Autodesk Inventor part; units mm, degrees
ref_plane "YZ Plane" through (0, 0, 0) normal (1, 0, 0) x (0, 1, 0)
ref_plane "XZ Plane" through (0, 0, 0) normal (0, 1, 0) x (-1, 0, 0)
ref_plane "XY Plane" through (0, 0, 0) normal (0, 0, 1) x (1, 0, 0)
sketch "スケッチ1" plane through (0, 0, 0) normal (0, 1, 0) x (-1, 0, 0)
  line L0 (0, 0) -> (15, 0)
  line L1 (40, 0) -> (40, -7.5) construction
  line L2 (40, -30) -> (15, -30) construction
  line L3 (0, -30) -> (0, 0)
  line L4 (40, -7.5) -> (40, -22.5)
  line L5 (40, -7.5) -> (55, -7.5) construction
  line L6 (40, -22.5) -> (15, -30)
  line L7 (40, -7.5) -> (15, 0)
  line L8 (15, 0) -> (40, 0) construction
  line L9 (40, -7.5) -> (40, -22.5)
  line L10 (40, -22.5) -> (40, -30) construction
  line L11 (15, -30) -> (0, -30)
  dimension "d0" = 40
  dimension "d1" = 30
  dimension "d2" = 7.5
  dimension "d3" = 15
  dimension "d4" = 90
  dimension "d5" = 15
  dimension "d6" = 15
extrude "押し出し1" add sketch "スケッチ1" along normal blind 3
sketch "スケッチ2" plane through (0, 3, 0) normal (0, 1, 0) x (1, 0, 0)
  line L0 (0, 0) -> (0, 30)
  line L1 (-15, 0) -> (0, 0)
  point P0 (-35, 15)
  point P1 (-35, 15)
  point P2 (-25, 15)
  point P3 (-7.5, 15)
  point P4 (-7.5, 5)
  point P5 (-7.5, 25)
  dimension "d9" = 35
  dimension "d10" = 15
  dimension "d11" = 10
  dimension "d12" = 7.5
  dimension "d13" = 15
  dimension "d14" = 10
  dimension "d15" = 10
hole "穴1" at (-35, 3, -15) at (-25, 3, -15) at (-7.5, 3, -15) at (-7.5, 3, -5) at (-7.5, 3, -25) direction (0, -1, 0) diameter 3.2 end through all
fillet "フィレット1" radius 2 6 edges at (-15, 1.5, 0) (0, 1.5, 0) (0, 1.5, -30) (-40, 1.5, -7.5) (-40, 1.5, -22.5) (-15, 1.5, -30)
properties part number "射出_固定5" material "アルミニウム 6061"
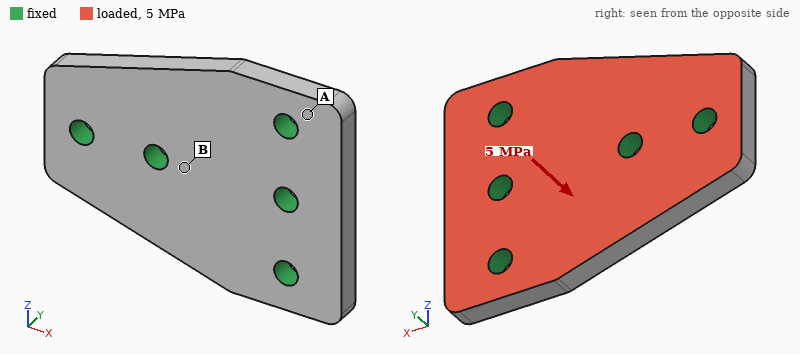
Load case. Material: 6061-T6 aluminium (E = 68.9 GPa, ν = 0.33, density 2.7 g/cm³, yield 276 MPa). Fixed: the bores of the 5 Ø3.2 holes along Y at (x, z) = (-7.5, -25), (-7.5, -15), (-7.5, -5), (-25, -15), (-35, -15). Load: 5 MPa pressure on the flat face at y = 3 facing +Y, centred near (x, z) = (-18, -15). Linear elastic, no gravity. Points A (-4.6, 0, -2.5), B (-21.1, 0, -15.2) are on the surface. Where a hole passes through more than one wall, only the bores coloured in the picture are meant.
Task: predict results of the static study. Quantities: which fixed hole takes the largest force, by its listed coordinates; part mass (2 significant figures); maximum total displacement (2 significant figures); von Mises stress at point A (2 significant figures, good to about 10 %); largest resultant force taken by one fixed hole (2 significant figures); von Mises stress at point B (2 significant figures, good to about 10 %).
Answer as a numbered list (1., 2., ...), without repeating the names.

1. (-25, -15)
2. 7.9 g
3. 46 µm
4. 32 MPa
5. 1.4 kN
6. 79 MPa
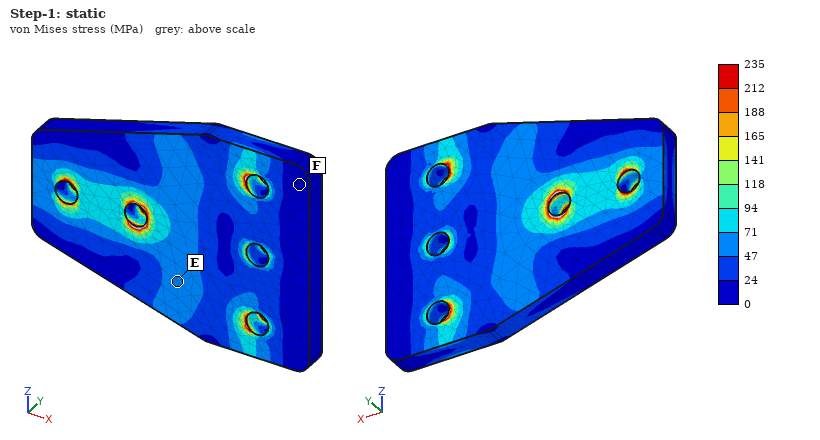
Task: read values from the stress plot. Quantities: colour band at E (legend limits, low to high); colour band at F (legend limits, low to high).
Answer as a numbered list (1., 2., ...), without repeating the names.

1. 47 to 71 MPa
2. 0 to 24 MPa
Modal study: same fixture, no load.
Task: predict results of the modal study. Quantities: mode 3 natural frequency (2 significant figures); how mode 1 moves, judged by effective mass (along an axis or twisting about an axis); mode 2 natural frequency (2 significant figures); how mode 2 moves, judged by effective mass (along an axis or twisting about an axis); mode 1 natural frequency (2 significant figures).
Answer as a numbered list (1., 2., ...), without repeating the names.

1. 38 kHz
2. twisting about X
3. 25 kHz
4. along Y
5. 23 kHz
